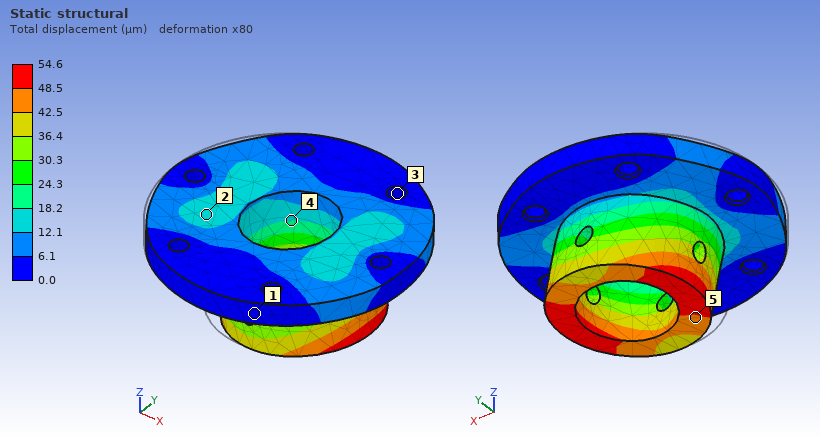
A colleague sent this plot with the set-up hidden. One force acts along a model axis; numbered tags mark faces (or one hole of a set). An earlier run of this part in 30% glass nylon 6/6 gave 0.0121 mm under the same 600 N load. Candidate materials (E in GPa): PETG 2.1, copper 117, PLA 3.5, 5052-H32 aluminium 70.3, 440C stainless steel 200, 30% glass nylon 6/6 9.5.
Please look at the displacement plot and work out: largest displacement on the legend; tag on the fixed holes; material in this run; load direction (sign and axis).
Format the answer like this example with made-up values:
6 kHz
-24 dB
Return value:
54.6 µm
3
PETG
+X
